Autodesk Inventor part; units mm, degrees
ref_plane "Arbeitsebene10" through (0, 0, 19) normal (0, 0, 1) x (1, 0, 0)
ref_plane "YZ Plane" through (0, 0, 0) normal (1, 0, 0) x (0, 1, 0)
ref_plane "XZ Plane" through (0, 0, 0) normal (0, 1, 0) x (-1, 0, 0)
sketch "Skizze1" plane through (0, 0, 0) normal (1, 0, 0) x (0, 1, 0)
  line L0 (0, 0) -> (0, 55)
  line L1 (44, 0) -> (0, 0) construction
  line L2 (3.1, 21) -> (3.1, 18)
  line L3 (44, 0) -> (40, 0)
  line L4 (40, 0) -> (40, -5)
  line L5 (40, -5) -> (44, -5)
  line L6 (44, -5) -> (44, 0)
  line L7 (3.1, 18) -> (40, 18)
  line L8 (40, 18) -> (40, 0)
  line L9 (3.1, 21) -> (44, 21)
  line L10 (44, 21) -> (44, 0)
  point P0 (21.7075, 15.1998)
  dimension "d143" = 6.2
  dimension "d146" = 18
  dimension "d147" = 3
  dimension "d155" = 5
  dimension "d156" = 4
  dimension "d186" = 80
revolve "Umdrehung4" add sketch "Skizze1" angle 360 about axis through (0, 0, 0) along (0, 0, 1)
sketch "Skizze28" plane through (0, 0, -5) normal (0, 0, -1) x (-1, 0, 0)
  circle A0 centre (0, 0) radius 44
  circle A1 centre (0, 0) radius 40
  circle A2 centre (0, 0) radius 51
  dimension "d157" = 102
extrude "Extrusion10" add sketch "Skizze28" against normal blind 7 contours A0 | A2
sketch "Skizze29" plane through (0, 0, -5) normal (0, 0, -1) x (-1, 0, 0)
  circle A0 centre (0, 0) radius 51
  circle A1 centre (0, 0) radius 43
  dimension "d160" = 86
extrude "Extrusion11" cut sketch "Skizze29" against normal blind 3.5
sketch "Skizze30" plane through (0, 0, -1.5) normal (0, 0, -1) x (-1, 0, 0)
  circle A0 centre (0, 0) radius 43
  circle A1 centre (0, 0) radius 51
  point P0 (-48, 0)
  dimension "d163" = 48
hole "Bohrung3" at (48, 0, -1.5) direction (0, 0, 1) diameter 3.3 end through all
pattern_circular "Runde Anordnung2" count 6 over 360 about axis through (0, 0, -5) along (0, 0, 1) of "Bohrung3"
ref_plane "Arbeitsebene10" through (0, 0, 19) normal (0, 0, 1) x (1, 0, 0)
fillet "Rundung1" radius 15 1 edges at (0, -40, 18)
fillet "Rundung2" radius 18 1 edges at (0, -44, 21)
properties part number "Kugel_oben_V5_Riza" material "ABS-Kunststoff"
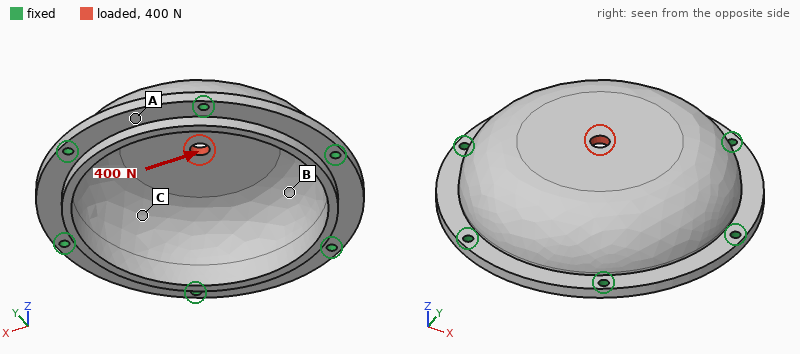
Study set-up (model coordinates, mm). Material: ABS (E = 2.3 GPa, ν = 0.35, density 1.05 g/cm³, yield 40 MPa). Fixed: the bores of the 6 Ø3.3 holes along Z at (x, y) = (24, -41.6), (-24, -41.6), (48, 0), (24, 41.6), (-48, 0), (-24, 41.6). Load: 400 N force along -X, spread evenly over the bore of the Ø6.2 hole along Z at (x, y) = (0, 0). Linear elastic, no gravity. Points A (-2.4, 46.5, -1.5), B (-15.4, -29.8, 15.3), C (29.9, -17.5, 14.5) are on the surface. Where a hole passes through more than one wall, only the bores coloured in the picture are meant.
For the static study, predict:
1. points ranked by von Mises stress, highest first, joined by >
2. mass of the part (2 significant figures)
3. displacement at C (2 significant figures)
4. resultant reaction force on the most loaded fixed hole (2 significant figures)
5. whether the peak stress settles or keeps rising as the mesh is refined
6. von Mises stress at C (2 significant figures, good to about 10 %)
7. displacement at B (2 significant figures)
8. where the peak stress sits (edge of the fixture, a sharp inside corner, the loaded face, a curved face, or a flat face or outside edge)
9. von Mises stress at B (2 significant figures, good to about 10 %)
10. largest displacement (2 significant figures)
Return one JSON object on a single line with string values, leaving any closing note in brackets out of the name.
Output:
{"points ranked by von Mises stress, highest first, joined by >": "B > C > A", "mass of the part": "44 g", "displacement at C": "0.040 mm", "resultant reaction force on the most loaded fixed hole": "84 N", "whether the peak stress settles or keeps rising as the mesh is refined": "keeps rising", "von Mises stress at C": "1.3 MPa", "displacement at B": "0.034 mm", "where the peak stress sits": "edge of the fixture", "von Mises stress at B": "1.9 MPa", "largest displacement": "0.10 mm"}
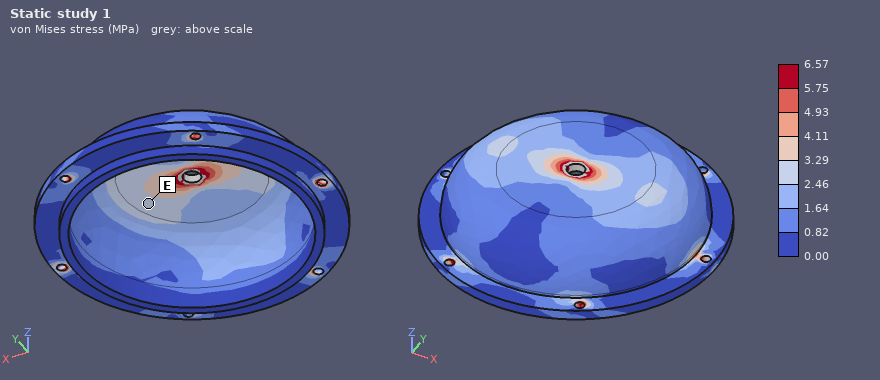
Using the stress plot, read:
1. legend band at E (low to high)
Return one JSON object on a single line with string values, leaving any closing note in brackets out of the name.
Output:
{"legend band at E": "2.46 to 3.29 MPa"}
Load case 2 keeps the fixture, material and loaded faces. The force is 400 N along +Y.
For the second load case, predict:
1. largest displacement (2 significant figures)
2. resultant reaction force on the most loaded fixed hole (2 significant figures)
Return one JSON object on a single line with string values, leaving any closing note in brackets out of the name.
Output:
{"largest displacement": "0.10 mm", "resultant reaction force on the most loaded fixed hole": "88 N"}
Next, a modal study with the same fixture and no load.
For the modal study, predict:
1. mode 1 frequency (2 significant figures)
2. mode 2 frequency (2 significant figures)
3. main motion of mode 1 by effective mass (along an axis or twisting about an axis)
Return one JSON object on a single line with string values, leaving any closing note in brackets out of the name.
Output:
{"mode 1 frequency": "1800 Hz", "mode 2 frequency": "3100 Hz", "main motion of mode 1 by effective mass": "along Z"}
